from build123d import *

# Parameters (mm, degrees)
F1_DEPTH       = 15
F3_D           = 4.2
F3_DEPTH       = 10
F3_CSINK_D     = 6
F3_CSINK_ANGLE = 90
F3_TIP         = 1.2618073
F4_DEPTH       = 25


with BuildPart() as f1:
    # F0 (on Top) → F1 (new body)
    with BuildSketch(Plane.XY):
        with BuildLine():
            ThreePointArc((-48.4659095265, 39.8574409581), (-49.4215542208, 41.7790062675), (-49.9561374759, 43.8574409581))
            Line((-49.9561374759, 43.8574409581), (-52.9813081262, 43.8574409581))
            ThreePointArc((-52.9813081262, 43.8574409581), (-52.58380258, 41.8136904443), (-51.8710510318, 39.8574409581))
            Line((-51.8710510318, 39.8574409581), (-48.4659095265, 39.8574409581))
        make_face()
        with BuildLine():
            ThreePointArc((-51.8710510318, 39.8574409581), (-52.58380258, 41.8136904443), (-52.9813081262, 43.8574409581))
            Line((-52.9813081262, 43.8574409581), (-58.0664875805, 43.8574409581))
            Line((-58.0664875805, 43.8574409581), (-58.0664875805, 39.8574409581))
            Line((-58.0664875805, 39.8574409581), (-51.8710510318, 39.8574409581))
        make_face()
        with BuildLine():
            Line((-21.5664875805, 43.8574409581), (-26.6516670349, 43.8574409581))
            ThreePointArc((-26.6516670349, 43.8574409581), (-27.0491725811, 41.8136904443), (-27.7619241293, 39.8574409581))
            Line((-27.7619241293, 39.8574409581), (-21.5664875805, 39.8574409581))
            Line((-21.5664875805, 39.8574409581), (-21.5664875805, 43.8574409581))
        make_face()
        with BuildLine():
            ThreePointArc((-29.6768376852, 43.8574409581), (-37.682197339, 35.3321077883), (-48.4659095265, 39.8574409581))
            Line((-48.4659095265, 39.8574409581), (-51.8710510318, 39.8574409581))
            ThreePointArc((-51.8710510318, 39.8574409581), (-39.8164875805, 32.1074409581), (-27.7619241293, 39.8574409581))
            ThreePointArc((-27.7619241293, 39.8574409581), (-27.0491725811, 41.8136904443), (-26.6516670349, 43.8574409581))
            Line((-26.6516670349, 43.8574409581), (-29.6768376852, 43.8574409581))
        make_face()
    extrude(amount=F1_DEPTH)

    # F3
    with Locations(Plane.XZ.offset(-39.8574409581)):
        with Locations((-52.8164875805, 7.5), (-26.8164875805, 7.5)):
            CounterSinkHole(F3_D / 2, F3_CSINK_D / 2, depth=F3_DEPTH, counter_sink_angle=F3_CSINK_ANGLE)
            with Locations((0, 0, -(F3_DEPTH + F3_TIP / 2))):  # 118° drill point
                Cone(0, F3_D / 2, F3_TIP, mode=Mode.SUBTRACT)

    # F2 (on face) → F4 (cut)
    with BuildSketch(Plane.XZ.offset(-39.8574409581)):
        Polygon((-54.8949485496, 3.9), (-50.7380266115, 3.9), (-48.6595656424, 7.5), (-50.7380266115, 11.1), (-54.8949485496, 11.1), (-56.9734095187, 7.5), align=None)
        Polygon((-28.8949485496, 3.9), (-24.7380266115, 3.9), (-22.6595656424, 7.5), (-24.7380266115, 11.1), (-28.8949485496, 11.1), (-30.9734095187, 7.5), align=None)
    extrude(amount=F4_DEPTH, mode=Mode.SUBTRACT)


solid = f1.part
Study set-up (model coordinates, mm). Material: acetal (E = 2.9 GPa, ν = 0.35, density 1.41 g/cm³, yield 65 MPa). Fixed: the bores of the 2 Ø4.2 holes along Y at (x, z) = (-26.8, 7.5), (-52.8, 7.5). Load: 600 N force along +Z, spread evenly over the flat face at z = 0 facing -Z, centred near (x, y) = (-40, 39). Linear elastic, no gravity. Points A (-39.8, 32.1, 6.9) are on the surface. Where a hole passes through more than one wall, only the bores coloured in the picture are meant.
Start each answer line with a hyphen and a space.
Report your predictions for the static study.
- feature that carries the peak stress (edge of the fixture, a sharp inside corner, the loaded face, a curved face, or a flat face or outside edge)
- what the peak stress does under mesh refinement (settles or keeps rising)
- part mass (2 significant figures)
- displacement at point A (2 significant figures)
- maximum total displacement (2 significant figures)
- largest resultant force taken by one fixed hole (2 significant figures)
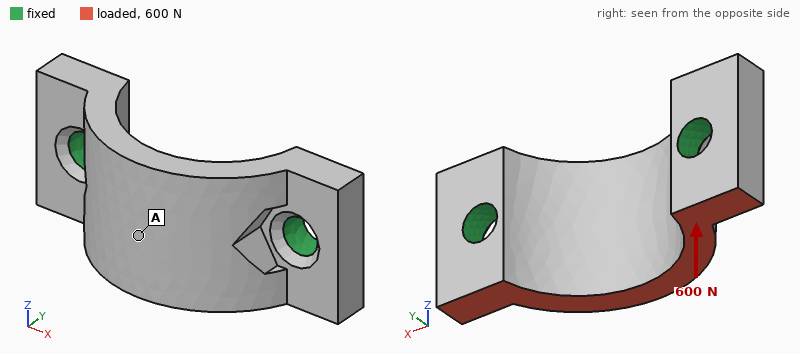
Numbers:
- edge of the fixture
- keeps rising
- 2.8 g
- 0.18 mm
- 0.23 mm
- 300 N
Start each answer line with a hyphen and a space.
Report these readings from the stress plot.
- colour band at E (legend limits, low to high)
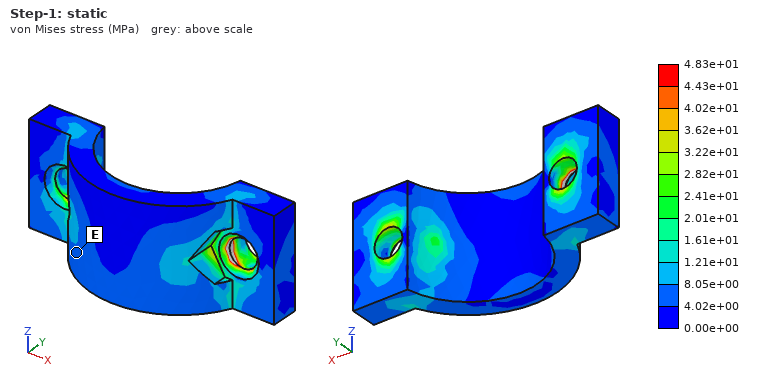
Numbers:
- 4.02e+00 to 8.05e+00 MPa
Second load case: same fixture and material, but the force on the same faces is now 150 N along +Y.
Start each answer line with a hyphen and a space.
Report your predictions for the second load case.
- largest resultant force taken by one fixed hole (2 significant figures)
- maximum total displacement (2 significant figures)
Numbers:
- 79 N
- 0.10 mm
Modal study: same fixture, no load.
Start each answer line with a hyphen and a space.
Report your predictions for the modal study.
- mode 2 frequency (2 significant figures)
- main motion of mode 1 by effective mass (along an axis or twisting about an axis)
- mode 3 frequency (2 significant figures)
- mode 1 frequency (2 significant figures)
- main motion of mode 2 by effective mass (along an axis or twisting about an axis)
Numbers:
- 8100 Hz
- along Z
- 9900 Hz
- 5400 Hz
- along X
